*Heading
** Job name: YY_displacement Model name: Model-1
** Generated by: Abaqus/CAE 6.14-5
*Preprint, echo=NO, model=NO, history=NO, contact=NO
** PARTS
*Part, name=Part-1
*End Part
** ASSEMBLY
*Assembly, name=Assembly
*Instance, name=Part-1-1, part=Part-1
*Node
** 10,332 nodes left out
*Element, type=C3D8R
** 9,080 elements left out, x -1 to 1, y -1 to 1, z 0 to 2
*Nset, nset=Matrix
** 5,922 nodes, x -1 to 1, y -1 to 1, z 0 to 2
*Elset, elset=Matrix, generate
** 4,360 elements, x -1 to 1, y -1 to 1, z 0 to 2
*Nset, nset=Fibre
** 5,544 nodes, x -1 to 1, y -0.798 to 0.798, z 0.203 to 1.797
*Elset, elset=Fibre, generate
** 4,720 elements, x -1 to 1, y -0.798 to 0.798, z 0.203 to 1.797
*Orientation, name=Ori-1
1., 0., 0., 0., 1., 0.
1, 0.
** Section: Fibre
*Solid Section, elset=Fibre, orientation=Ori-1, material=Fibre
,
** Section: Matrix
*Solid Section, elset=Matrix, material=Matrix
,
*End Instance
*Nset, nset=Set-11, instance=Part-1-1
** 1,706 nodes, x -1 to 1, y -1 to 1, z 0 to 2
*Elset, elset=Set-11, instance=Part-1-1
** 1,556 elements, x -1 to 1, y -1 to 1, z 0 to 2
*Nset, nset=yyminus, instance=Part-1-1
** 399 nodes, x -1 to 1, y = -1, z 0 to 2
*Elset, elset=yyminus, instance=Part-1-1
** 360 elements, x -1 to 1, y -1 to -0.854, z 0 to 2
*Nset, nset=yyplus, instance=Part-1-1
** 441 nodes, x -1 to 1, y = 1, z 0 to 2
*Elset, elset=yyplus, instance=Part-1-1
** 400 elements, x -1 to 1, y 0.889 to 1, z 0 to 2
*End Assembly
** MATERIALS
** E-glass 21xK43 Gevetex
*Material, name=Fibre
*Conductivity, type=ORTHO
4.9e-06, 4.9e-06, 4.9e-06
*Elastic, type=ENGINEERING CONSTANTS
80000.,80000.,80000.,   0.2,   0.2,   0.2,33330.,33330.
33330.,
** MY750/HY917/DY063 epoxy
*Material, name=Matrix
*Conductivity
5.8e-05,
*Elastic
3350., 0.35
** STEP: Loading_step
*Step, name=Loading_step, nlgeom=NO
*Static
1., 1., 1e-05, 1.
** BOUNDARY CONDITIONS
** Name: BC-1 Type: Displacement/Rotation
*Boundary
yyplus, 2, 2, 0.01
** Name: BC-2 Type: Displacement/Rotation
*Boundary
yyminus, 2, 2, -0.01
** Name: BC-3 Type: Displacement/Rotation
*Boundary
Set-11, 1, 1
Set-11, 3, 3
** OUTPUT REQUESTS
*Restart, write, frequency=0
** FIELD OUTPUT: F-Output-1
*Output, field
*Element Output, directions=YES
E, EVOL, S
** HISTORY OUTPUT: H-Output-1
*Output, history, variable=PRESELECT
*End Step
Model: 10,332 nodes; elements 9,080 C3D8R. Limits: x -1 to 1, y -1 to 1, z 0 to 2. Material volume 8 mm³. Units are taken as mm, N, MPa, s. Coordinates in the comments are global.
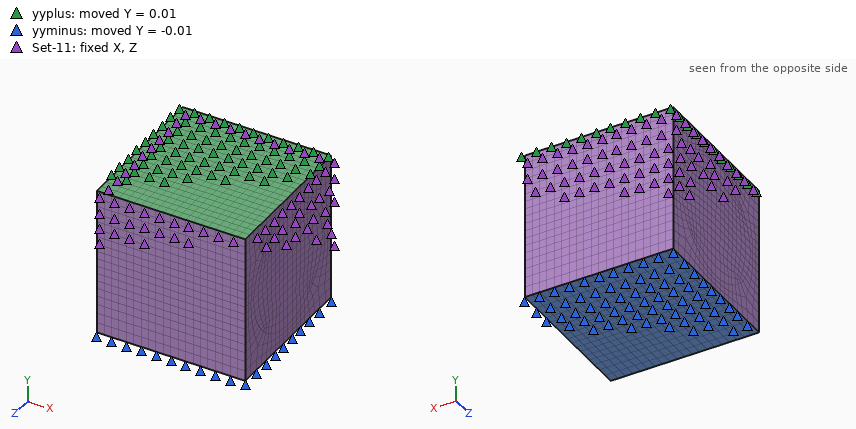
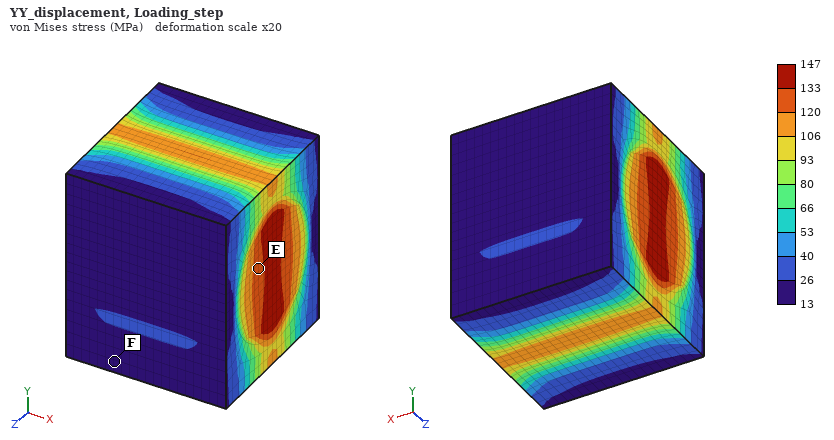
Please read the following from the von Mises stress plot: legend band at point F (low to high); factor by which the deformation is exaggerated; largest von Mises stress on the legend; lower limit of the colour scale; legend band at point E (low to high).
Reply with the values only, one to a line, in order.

13 to 26 MPa
20
147 MPa
13 MPa
120 to 133 MPa
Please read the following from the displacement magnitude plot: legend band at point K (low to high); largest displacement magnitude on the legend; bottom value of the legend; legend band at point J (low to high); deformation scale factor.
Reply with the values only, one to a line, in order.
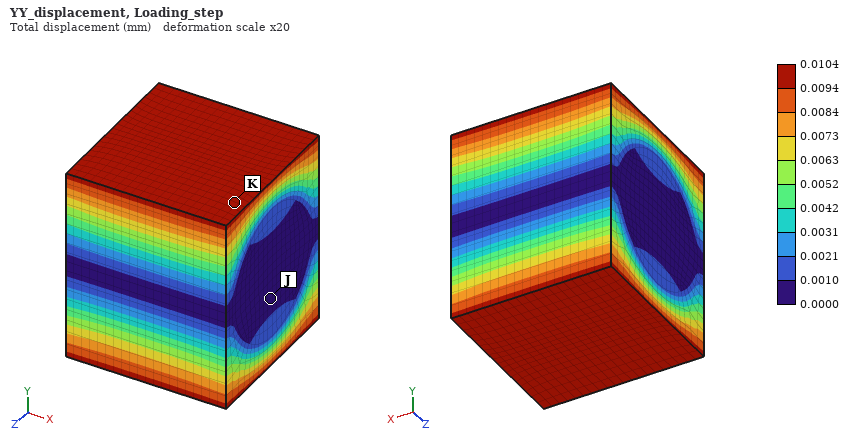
0.0094 to 0.0104 mm
0.0104 mm
0.0000 mm
0.0000 to 0.0010 mm
20
